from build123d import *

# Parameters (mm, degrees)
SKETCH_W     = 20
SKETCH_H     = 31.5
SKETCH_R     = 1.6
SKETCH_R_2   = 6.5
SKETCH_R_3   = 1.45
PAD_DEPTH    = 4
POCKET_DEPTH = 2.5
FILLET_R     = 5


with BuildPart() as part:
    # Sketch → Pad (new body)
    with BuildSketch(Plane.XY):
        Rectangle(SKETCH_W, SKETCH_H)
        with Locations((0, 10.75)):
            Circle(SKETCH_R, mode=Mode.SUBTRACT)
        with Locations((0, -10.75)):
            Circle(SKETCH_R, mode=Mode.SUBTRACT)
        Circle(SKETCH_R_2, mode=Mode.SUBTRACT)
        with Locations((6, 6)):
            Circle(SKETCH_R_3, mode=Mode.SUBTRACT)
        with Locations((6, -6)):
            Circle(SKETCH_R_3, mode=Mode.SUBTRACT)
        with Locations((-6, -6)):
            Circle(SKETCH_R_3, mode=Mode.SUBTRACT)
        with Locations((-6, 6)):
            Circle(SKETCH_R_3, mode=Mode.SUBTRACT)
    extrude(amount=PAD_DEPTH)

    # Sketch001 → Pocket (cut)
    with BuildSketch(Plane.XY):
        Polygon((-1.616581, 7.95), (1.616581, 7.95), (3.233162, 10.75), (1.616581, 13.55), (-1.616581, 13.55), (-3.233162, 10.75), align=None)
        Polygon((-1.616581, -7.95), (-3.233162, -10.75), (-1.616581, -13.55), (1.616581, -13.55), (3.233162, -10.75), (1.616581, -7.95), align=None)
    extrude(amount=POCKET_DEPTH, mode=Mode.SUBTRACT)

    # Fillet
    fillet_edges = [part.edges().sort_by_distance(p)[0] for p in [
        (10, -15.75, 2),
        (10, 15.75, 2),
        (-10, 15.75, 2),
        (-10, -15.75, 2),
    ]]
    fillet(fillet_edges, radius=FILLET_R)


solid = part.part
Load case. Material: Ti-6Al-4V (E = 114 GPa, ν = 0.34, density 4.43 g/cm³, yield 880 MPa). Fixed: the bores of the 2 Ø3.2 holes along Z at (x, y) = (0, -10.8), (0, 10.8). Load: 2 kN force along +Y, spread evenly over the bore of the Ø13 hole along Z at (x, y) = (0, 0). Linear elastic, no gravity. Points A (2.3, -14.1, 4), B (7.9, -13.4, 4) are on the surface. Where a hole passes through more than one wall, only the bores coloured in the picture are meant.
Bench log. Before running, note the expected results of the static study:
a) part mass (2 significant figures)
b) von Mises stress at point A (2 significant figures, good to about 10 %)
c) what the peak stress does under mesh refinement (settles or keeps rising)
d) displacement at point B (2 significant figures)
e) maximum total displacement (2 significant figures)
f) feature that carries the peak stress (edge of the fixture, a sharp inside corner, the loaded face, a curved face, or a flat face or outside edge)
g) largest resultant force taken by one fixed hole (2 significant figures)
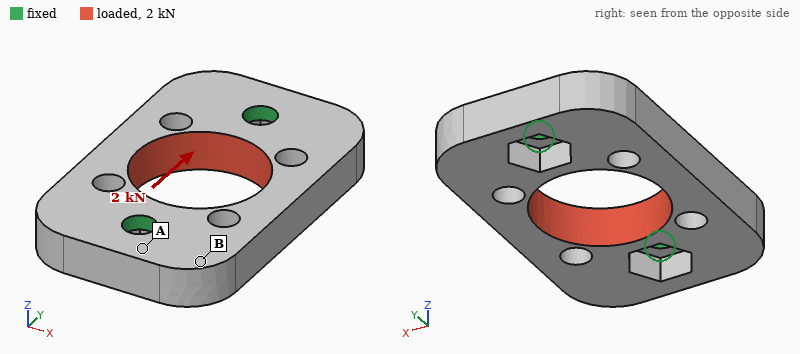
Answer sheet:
7.3 g
40 MPa
keeps rising
4.4 µm
7.6 µm
edge of the fixture
1.0 kN
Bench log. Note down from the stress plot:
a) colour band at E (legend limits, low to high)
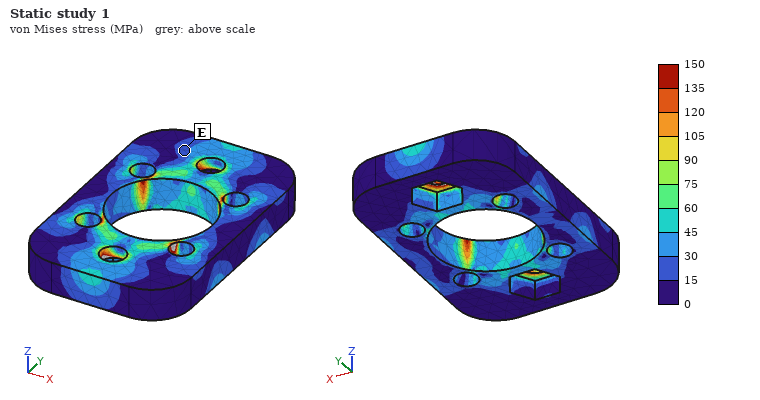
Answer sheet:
15 to 30 MPa
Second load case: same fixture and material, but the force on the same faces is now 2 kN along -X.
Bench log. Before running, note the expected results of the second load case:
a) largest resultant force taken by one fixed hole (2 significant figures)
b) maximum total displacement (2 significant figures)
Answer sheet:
1.0 kN
25 µm
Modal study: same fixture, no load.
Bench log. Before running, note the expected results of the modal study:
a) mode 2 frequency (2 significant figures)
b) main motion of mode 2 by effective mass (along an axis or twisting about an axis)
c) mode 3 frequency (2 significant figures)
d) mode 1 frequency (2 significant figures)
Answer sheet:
18 kHz
along Z
19 kHz
11 kHz
